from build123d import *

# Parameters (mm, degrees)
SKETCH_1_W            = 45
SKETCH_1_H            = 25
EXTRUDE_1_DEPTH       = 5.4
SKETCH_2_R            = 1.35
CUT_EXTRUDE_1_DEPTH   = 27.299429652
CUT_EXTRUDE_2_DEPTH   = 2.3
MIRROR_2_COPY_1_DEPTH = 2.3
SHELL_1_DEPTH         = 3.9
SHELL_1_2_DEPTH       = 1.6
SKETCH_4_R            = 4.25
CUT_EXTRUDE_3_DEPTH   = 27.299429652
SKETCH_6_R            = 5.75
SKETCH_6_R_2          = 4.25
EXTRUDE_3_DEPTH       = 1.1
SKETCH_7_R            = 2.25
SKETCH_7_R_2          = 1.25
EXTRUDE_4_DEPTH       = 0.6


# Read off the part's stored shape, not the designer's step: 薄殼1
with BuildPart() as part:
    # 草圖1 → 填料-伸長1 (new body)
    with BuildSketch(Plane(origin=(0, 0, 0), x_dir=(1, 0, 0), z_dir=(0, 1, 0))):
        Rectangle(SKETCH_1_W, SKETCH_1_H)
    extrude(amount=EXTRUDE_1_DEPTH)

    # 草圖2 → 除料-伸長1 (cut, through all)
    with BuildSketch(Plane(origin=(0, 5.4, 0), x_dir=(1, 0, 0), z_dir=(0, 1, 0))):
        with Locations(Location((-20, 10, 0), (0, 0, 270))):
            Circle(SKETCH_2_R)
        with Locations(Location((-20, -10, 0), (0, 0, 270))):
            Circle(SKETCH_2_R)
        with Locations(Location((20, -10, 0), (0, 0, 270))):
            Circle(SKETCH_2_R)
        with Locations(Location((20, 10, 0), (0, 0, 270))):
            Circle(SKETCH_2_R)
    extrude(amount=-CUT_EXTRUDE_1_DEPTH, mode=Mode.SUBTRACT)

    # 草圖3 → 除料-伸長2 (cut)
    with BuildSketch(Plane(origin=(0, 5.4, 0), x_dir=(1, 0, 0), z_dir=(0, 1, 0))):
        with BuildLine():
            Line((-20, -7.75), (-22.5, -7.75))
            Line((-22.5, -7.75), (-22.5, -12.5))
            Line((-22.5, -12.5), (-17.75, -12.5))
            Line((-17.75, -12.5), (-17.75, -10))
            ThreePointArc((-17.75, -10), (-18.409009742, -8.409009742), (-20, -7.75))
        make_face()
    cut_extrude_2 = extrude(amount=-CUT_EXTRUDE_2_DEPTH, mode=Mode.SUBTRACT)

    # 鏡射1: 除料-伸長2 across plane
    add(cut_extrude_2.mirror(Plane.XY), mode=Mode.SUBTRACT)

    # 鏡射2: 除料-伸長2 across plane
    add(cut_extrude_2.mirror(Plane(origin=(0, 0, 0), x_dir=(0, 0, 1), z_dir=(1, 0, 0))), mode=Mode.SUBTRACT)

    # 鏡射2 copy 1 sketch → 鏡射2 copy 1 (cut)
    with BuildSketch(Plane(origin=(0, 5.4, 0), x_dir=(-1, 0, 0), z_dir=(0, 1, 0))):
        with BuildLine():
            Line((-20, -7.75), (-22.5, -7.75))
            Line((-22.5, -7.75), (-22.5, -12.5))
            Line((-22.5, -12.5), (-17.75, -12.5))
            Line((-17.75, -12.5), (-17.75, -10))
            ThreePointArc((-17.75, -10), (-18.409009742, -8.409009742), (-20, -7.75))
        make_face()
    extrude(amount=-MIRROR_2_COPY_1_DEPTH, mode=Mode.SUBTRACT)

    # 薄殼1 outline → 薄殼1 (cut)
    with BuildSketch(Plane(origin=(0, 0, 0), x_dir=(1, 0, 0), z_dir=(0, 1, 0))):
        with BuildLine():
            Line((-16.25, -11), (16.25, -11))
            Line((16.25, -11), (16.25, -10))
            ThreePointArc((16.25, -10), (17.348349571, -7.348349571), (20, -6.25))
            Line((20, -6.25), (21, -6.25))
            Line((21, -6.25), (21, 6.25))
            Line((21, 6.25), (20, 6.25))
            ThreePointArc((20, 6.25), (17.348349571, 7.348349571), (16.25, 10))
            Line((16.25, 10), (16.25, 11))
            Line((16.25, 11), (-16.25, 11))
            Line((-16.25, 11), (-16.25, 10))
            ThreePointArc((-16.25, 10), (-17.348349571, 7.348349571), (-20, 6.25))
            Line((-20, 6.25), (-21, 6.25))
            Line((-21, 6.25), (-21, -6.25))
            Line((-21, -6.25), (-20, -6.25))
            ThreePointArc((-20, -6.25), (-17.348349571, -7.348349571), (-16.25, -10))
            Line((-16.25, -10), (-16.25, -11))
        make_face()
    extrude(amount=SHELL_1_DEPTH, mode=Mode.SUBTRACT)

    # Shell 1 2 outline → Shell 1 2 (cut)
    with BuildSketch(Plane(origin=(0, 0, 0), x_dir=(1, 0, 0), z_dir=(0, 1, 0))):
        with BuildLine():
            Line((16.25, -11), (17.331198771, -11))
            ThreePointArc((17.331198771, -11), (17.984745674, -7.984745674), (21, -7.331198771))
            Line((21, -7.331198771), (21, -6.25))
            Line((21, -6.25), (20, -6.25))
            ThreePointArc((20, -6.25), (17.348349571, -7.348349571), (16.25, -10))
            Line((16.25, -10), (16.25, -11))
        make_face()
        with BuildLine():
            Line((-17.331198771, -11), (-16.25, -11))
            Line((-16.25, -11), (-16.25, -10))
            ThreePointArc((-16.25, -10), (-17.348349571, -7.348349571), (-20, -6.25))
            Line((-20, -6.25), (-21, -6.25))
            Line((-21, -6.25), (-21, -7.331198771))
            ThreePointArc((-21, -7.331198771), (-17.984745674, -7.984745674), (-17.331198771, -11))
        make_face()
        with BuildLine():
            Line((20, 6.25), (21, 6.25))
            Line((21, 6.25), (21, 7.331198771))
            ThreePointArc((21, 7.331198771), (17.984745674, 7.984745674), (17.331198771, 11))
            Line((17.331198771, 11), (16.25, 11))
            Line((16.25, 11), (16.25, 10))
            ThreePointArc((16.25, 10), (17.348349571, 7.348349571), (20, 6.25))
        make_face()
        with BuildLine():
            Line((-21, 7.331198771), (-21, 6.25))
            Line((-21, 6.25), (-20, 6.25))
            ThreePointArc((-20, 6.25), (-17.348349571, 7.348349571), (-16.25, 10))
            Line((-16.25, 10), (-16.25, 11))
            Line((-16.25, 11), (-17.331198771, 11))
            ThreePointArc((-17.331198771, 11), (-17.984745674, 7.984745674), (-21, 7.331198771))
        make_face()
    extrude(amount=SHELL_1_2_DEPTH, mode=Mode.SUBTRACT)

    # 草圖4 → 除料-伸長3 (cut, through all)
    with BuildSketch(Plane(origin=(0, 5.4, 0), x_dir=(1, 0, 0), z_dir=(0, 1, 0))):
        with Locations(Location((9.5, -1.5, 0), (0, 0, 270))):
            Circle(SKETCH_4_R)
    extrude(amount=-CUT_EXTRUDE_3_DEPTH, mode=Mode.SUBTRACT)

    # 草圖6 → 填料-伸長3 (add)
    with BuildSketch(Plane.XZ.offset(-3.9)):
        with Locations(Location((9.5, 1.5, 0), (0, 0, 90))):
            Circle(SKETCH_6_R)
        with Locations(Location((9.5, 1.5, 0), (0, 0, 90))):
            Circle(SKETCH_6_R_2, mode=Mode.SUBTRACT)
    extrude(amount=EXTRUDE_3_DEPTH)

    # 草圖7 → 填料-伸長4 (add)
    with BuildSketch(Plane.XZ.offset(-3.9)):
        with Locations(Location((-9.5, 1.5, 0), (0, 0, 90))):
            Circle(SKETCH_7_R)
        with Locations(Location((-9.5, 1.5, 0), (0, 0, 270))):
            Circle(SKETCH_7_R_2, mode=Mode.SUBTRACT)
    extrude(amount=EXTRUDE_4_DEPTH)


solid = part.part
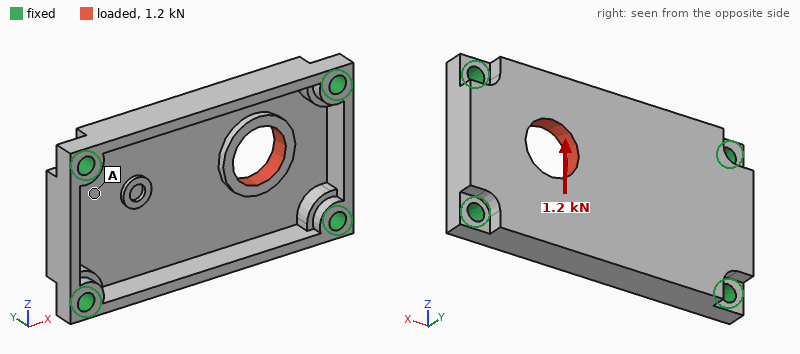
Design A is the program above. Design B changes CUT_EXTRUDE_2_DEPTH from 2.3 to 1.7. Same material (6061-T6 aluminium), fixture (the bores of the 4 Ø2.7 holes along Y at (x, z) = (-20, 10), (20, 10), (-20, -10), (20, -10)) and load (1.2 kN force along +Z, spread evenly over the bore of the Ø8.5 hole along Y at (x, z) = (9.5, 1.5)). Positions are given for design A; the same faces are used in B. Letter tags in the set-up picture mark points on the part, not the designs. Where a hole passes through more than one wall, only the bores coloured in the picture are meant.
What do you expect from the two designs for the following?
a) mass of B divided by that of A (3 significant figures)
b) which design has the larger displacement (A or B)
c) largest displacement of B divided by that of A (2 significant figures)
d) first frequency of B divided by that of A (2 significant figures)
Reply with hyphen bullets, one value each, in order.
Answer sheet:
- 1.01
- A
- 0.92
- 1.0
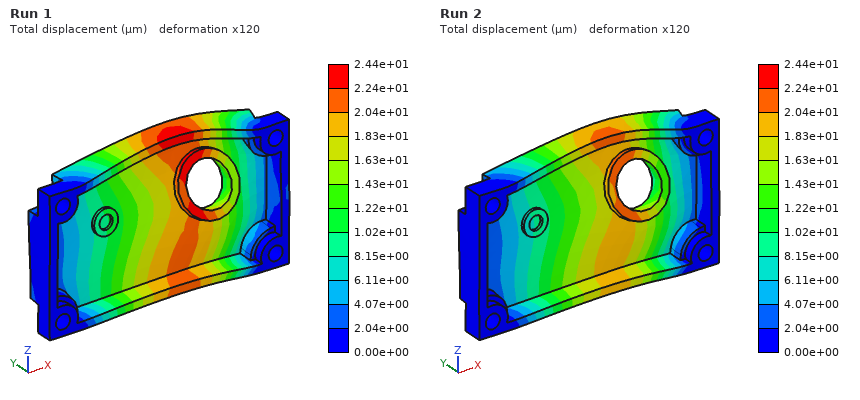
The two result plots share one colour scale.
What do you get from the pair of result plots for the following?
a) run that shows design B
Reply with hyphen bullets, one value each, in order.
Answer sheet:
- Run 2
